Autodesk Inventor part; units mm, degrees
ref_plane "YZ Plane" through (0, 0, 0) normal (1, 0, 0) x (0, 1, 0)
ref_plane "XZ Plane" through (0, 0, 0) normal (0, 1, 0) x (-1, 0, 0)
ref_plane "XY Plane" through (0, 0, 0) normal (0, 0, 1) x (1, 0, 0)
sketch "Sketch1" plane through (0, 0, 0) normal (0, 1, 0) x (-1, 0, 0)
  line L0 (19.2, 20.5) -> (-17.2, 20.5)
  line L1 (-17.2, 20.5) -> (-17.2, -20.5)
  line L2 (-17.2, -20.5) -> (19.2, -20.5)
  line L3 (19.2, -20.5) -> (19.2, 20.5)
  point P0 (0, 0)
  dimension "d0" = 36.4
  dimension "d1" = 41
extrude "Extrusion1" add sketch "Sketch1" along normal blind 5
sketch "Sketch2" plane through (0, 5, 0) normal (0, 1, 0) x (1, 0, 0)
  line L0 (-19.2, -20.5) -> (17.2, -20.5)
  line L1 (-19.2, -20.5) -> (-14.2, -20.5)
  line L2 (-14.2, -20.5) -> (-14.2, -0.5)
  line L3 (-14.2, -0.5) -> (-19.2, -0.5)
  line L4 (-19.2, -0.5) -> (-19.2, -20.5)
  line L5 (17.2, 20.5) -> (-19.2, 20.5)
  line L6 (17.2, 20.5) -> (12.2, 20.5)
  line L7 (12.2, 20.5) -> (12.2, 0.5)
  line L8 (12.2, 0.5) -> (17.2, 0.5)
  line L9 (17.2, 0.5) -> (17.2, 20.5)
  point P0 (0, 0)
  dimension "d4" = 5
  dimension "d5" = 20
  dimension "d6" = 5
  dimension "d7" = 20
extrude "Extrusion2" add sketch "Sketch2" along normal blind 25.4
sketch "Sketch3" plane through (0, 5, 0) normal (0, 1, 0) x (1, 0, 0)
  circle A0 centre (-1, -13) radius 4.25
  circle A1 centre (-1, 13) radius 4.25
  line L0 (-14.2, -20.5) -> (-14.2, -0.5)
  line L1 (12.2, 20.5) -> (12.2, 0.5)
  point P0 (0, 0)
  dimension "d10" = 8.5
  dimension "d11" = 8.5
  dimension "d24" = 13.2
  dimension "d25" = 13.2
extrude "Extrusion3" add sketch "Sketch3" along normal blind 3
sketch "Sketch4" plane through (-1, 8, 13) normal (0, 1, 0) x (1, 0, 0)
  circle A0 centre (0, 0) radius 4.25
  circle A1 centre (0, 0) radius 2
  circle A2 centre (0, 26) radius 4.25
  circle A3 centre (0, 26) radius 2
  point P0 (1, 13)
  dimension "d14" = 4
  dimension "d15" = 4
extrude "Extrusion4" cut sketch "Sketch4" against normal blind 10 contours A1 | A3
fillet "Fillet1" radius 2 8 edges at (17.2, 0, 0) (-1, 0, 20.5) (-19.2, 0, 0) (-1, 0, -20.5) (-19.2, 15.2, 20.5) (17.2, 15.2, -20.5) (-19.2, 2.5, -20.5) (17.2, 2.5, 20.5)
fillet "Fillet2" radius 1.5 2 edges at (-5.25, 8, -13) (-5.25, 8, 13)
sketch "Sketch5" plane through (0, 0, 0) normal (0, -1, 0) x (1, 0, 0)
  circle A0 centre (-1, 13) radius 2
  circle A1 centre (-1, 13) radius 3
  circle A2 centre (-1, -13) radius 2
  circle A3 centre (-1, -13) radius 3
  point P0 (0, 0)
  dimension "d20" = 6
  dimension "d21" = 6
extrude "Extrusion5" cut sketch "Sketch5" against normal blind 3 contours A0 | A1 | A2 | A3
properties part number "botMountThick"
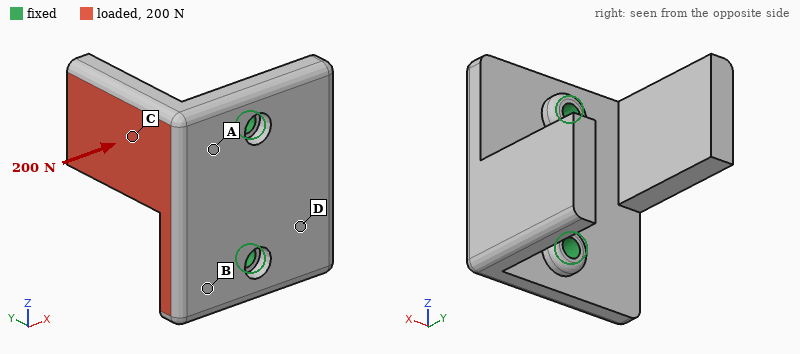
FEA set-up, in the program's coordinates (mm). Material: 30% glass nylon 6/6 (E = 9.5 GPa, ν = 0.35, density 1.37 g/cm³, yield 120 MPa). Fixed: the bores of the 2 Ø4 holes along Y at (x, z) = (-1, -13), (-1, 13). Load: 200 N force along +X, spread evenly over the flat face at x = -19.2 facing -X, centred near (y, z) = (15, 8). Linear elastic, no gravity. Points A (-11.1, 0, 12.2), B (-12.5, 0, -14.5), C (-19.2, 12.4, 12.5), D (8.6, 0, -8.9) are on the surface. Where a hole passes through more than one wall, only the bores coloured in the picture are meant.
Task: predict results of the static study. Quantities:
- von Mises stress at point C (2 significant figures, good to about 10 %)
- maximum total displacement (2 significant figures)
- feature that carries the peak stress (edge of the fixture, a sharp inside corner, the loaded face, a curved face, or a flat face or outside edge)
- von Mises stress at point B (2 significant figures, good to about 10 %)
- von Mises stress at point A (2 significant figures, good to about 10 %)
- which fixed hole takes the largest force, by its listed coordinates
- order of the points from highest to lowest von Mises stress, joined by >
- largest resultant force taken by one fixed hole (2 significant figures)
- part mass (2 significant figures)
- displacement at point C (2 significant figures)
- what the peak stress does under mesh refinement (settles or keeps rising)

11 MPa
0.63 mm
a sharp inside corner
7.0 MPa
19 MPa
(-1, 13)
A > C > B > D
160 N
17 g
0.25 mm
keeps rising
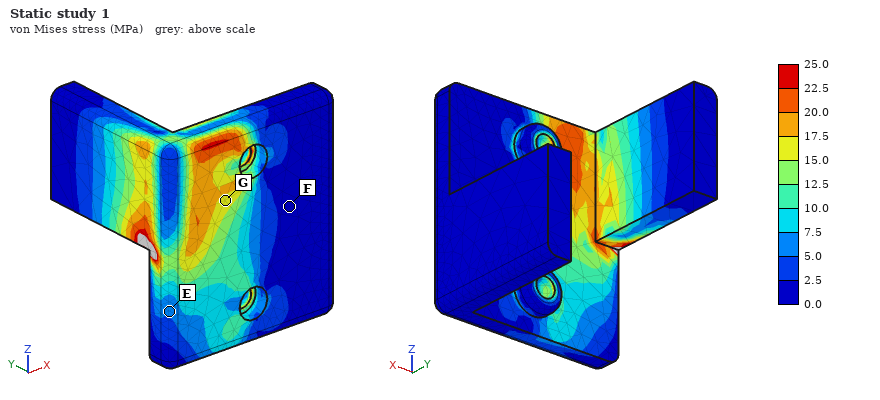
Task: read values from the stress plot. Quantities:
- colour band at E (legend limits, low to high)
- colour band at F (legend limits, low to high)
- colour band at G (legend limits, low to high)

5.0 to 7.5 MPa
0.0 to 2.5 MPa
15.0 to 17.5 MPa
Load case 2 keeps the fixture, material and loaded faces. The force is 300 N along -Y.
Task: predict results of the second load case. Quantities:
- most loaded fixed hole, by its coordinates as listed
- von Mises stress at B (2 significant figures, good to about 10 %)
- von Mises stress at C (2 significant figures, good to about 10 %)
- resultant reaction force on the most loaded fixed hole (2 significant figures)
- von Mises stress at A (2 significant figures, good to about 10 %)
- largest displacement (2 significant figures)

(-1, 13)
11 MPa
5.9 MPa
240 N
16 MPa
0.69 mm
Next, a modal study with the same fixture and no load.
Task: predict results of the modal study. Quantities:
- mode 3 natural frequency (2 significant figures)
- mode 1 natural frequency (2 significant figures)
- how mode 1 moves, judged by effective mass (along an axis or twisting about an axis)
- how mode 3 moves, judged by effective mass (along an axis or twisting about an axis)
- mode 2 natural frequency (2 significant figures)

2600 Hz
1500 Hz
along X
twisting about Y
1700 Hz
